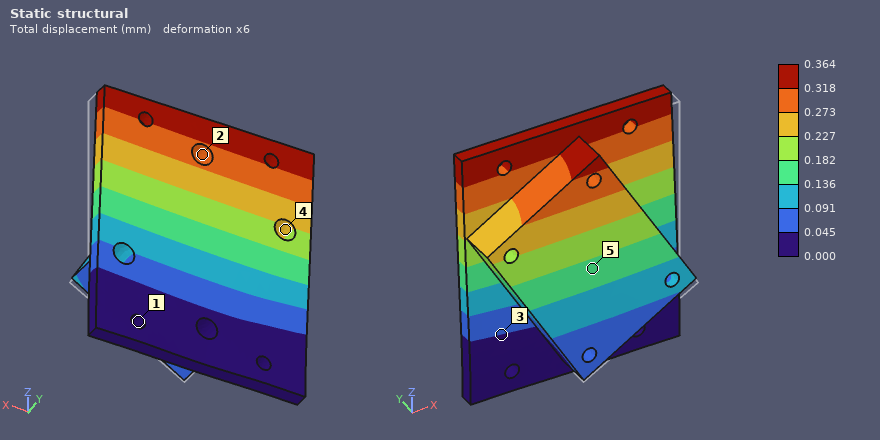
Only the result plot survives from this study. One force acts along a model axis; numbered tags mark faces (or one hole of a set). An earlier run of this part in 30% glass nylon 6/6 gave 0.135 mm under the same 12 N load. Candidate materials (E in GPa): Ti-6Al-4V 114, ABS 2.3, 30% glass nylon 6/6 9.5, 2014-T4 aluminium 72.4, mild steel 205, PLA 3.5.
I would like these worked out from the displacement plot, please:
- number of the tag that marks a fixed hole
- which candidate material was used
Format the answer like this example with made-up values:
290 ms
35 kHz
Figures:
1
PLA
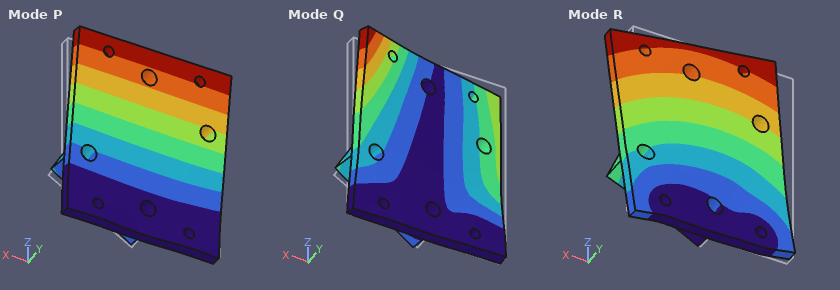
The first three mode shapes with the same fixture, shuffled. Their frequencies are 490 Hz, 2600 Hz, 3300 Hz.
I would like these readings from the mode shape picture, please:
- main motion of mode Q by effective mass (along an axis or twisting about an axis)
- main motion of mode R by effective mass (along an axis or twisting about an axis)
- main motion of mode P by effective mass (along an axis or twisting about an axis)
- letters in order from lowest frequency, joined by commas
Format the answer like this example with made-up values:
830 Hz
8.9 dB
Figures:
twisting about Z
along X
along Y
P, Q, R
